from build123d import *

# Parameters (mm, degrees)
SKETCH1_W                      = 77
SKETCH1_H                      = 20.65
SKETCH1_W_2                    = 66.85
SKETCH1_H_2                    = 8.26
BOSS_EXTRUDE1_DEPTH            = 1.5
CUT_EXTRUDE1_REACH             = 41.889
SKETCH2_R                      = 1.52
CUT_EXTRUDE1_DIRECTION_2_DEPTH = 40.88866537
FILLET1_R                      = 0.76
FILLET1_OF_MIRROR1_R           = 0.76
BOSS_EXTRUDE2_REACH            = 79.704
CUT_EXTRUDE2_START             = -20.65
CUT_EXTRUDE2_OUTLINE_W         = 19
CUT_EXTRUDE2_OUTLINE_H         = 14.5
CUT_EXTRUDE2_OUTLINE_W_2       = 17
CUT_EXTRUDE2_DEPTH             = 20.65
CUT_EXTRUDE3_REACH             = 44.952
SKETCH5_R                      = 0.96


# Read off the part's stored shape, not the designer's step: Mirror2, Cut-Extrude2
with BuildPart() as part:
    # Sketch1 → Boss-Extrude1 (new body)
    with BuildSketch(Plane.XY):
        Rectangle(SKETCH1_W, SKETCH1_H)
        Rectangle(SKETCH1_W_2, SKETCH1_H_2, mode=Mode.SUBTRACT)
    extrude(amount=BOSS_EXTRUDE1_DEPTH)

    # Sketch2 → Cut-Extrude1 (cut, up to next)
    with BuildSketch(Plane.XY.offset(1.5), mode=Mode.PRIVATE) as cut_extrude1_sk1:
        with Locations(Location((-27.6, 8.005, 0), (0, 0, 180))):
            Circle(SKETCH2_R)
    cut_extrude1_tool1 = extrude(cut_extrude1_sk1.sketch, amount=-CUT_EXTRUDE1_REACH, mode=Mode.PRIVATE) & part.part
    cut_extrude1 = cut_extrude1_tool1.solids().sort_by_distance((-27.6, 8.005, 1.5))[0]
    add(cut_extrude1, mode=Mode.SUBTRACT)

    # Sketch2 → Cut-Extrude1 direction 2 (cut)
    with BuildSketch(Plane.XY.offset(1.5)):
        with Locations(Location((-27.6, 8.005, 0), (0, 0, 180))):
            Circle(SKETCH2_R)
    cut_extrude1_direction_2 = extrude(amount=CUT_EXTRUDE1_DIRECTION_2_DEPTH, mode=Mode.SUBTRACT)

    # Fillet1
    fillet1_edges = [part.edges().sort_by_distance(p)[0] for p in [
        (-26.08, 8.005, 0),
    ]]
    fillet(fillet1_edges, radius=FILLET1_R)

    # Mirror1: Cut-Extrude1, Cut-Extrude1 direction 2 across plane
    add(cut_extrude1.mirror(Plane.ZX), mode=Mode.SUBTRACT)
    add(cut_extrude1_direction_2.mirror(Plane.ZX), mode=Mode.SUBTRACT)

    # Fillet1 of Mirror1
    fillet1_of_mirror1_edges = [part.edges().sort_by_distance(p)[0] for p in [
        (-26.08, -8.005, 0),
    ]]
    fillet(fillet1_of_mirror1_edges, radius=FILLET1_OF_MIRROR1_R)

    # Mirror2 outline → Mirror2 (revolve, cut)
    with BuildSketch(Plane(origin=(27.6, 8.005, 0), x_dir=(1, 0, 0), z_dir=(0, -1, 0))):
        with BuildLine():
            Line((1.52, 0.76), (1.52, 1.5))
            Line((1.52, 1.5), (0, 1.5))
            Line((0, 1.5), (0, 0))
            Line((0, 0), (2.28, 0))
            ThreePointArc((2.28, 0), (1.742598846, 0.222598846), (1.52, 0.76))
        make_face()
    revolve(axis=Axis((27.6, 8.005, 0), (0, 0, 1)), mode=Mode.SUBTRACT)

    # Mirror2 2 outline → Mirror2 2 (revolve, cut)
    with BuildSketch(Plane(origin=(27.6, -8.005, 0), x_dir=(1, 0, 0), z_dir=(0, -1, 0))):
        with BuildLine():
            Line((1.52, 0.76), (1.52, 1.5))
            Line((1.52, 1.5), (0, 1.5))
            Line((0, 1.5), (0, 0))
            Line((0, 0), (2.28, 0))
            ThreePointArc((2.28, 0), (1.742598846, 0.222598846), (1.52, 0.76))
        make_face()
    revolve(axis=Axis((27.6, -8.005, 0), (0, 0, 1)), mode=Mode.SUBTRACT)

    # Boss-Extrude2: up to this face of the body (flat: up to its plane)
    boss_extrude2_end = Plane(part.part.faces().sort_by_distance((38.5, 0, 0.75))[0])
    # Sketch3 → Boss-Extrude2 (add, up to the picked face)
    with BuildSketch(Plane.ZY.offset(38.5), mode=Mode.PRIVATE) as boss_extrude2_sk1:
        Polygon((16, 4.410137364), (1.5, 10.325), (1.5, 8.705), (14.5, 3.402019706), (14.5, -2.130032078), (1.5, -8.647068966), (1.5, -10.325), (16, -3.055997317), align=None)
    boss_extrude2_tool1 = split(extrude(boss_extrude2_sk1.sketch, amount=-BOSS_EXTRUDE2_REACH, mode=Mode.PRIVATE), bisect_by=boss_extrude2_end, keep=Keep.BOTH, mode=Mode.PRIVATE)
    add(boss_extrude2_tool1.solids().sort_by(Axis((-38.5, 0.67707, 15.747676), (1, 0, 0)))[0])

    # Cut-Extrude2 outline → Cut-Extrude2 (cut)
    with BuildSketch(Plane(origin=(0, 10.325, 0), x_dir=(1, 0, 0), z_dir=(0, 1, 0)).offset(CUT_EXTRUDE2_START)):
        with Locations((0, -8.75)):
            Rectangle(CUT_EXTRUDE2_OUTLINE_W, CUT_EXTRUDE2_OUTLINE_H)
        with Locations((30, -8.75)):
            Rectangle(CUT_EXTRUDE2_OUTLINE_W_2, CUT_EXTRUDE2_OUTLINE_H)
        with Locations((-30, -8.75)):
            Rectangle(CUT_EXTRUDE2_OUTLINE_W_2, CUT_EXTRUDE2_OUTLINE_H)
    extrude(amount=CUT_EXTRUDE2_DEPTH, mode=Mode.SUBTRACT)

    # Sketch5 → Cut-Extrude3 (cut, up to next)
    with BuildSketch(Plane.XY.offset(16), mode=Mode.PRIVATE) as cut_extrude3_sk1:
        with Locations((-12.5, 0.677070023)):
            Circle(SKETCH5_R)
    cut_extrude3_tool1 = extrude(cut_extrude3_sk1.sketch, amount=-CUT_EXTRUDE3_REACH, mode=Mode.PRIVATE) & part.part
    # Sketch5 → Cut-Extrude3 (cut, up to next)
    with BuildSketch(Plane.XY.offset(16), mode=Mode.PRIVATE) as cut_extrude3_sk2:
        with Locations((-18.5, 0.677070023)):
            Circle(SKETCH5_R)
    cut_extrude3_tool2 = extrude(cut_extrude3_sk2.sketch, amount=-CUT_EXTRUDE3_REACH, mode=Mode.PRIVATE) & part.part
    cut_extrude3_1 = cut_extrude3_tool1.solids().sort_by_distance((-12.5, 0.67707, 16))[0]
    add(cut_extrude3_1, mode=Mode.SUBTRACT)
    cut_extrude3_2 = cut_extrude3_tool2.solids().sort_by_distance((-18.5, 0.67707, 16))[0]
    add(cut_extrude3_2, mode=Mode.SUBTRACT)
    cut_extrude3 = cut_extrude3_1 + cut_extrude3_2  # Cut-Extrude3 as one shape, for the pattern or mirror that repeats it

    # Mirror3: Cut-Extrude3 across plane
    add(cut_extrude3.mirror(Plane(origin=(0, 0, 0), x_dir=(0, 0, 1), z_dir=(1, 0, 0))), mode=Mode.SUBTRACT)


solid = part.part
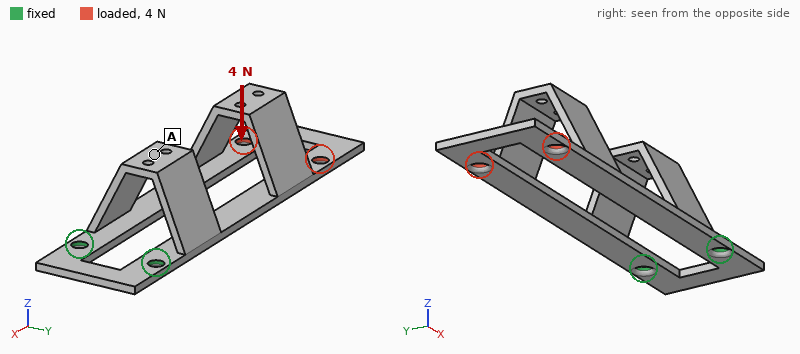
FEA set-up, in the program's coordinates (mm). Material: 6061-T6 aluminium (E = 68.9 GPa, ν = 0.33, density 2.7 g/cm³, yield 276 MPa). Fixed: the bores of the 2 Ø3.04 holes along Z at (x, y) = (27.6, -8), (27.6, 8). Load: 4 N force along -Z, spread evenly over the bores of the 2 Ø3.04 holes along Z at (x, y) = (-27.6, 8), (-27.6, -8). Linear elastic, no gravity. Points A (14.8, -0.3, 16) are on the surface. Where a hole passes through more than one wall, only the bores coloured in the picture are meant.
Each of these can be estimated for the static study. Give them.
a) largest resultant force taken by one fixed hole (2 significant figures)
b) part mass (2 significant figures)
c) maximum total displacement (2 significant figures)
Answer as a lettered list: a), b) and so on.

a) 3.1 N
b) 7.6 g
c) 0.84 mm
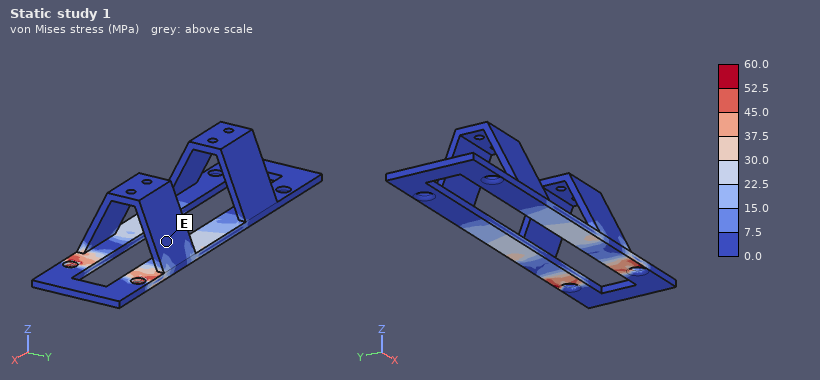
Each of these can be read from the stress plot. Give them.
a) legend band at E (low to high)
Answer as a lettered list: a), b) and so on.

a) 0.0 to 7.5 MPa
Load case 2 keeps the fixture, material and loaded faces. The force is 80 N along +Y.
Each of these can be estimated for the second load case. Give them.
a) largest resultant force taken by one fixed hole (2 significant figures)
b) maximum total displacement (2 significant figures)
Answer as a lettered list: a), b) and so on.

a) 160 N
b) 0.46 mm
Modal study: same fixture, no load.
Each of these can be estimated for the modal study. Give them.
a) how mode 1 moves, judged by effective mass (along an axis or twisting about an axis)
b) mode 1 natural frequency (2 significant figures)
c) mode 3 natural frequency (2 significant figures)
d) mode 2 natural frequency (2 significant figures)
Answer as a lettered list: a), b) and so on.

a) along Z
b) 250 Hz
c) 1300 Hz
d) 1300 Hz
